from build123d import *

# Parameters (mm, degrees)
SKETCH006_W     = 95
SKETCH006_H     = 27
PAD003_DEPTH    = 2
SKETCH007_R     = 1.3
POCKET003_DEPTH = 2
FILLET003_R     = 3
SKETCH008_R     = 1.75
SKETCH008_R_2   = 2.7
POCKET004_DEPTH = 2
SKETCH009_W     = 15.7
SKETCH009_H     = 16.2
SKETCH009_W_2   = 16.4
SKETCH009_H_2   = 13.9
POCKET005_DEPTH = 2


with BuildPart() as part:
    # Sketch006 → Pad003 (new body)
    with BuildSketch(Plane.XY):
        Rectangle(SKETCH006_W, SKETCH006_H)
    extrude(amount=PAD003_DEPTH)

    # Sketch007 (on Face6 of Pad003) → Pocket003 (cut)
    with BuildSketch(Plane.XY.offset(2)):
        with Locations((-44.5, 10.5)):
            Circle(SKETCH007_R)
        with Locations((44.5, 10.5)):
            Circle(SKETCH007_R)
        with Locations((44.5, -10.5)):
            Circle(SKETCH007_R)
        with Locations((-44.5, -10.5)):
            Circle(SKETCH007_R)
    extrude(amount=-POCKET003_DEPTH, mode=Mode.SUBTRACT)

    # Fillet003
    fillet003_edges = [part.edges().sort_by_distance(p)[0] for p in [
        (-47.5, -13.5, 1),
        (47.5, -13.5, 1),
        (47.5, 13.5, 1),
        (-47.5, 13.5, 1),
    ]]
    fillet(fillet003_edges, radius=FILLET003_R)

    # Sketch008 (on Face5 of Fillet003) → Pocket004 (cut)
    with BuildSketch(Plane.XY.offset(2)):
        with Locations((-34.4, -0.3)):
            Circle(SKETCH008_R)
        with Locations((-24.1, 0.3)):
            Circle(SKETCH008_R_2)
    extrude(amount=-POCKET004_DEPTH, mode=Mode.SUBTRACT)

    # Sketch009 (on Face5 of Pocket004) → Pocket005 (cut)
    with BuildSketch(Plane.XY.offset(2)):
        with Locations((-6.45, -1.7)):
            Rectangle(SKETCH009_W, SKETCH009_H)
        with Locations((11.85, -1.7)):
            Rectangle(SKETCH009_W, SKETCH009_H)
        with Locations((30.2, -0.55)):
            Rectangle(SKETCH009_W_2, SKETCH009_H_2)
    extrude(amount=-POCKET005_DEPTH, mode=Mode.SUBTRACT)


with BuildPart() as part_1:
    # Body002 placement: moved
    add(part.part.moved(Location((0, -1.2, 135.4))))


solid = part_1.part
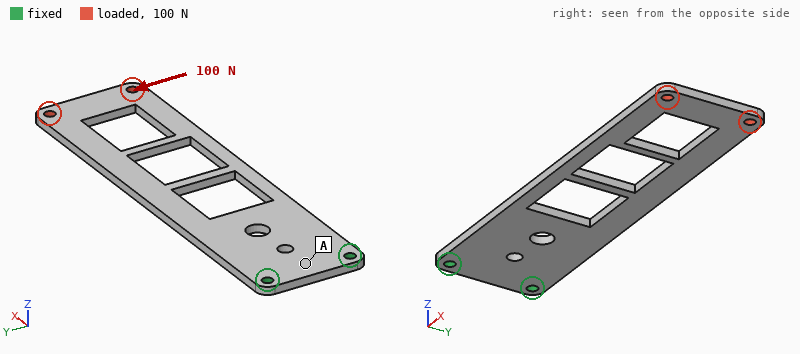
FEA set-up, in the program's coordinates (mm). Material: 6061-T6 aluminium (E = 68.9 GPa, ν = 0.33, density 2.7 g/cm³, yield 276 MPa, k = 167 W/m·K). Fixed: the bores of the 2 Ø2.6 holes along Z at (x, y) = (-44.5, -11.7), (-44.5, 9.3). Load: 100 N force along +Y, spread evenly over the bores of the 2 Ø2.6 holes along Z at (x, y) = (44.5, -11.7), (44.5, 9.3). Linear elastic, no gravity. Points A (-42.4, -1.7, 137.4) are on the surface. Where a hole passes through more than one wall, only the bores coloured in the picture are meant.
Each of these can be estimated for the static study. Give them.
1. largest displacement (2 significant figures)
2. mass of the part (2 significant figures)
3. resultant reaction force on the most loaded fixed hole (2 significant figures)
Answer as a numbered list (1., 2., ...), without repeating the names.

1. 0.34 mm
2. 9.5 g
3. 420 N
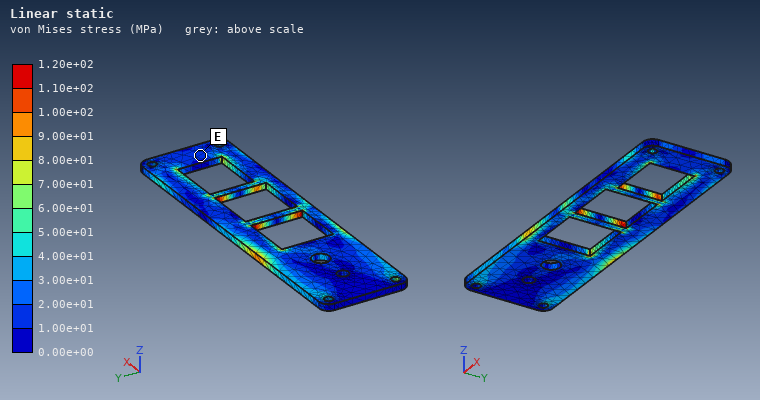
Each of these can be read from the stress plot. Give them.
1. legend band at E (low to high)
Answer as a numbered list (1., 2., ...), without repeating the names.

1. 1.00e+01 to 2.00e+01 MPa
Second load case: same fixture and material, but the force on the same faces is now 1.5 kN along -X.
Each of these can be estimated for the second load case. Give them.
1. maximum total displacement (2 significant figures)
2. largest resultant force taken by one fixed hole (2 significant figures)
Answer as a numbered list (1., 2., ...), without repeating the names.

1. 95 µm
2. 770 N
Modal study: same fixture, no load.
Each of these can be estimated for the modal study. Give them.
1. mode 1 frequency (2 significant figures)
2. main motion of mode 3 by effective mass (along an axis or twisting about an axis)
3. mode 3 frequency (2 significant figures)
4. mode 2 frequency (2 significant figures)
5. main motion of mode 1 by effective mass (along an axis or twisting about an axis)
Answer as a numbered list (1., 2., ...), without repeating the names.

1. 200 Hz
2. along Z
3. 1100 Hz
4. 1100 Hz
5. along Z
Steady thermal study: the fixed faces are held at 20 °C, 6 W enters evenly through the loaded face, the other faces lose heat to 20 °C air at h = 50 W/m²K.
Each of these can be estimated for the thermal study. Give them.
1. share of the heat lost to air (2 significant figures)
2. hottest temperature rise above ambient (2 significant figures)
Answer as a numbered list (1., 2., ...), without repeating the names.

1. 72 %
2. 56 K
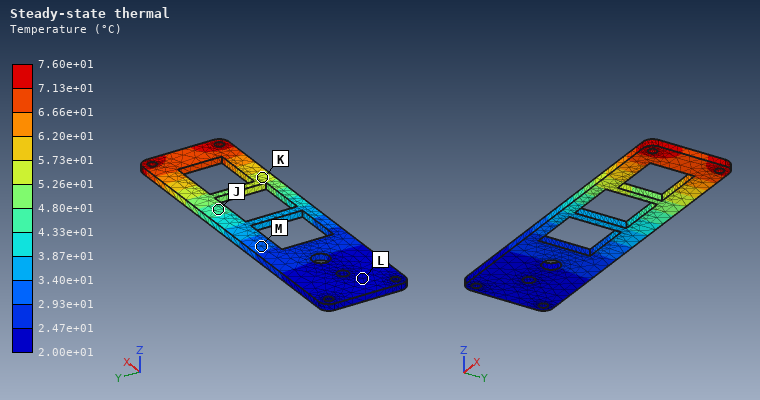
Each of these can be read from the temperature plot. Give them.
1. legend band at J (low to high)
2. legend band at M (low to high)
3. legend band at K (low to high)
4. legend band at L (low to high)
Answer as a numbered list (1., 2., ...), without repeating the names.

1. 4.33e+01 to 4.80e+01 °C
2. 2.93e+01 to 3.40e+01 °C
3. 5.26e+01 to 5.73e+01 °C
4. 2.00e+01 to 2.47e+01 °C
